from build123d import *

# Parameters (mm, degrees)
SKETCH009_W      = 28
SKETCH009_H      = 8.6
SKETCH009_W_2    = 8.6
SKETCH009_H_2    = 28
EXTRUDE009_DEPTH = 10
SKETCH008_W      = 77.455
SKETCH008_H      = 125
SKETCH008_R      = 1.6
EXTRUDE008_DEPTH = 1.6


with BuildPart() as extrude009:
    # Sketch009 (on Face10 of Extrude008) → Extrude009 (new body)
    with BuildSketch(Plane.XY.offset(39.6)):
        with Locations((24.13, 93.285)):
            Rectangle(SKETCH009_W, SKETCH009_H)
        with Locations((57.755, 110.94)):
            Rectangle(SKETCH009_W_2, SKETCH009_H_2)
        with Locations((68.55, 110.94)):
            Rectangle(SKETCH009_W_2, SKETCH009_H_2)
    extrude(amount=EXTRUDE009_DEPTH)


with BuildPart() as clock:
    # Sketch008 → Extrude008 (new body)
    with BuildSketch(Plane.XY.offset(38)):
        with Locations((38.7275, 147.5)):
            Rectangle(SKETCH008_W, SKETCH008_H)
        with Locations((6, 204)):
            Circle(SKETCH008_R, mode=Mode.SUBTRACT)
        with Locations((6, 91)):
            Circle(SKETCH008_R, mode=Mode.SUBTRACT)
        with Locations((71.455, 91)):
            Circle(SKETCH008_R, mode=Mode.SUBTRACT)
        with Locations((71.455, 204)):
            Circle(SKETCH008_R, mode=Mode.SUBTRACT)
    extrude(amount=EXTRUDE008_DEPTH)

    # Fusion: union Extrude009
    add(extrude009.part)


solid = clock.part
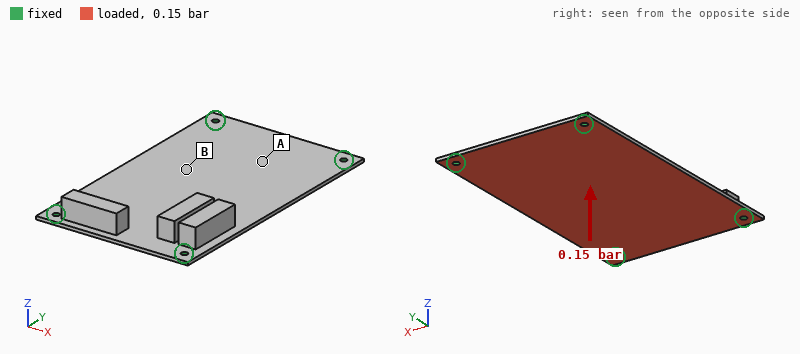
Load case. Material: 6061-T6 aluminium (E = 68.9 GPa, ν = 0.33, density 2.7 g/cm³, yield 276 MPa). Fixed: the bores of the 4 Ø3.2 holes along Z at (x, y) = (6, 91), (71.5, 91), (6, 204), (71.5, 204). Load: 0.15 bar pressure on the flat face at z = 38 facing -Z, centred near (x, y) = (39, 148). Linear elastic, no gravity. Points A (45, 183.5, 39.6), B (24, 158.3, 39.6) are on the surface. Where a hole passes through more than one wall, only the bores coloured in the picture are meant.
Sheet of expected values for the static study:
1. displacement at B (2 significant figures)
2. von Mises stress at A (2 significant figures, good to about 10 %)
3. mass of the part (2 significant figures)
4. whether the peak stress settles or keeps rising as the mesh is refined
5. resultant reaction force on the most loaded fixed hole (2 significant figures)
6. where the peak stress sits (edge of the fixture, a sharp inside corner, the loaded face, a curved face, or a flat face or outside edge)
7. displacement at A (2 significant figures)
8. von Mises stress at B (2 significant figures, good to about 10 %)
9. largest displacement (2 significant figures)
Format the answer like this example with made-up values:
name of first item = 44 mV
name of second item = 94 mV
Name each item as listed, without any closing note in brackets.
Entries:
displacement at B = 0.33 mm
von Mises stress at A = 8.3 MPa
mass of the part = 61 g
whether the peak stress settles or keeps rising as the mesh is refined = keeps rising
resultant reaction force on the most loaded fixed hole = 40 N
where the peak stress sits = edge of the fixture
displacement at A = 0.18 mm
von Mises stress at B = 17 MPa
largest displacement = 0.35 mm
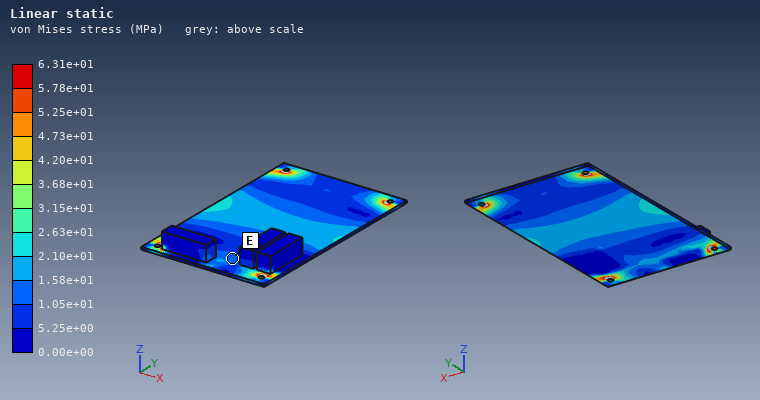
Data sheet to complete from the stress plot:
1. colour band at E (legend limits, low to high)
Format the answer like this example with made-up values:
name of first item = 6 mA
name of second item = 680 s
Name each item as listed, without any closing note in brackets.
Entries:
colour band at E = 1.05e+01 to 1.58e+01 MPa
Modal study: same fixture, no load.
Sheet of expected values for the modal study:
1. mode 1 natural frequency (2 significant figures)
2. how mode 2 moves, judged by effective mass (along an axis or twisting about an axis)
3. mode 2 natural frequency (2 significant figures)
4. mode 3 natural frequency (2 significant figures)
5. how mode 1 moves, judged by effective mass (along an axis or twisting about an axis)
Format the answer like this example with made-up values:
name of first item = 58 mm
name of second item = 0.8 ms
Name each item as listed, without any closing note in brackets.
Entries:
mode 1 natural frequency = 540 Hz
how mode 2 moves, judged by effective mass = twisting about Y
mode 2 natural frequency = 970 Hz
mode 3 natural frequency = 1400 Hz
how mode 1 moves, judged by effective mass = along Z
